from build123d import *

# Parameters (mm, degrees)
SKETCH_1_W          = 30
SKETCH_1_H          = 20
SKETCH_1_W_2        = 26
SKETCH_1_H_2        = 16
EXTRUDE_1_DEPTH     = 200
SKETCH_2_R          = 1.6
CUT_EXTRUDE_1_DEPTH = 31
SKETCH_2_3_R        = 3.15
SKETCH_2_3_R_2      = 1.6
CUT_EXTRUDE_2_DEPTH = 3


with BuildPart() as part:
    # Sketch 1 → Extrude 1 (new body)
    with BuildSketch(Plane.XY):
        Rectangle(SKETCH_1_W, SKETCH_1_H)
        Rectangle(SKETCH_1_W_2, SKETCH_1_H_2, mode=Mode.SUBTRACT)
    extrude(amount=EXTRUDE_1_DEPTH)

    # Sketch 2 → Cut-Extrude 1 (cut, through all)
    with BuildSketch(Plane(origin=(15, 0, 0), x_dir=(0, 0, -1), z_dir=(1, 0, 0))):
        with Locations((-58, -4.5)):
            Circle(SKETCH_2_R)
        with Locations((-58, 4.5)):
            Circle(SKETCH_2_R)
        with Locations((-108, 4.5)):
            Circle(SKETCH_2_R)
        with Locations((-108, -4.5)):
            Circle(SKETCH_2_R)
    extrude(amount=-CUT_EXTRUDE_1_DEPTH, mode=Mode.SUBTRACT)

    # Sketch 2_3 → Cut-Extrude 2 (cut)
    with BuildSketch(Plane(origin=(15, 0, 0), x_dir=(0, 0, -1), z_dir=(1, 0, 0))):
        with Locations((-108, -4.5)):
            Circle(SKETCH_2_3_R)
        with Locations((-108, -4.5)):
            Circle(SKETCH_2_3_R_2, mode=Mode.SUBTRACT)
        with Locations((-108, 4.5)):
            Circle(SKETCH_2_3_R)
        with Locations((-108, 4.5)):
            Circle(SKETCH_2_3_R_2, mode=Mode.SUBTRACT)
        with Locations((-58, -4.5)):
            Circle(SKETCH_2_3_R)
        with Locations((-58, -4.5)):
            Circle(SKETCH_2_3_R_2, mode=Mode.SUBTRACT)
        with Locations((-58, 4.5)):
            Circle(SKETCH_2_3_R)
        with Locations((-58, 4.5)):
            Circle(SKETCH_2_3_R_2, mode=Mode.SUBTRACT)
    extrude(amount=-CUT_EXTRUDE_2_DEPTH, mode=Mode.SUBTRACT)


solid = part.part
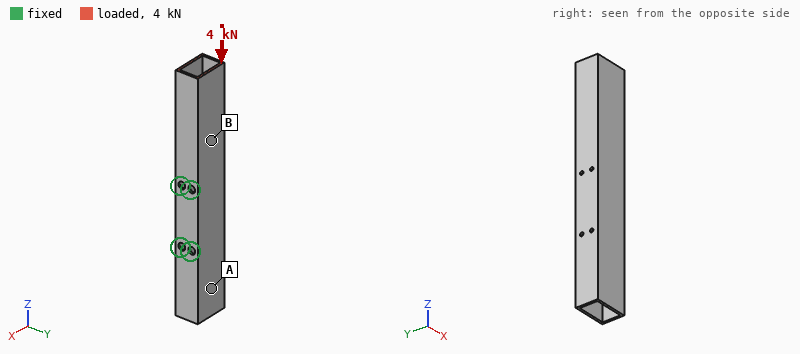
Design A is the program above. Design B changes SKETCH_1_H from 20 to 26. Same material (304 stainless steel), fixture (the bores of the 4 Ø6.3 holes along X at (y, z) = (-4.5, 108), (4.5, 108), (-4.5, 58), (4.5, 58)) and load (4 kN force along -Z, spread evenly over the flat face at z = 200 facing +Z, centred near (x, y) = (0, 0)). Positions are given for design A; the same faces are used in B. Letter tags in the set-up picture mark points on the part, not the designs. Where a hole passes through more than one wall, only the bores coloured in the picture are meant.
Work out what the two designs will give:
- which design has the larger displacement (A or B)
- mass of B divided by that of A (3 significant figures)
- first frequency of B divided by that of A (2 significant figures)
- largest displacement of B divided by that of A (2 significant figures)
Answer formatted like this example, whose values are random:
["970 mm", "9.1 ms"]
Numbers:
["A", "1.99", "1.0", "0.56"]
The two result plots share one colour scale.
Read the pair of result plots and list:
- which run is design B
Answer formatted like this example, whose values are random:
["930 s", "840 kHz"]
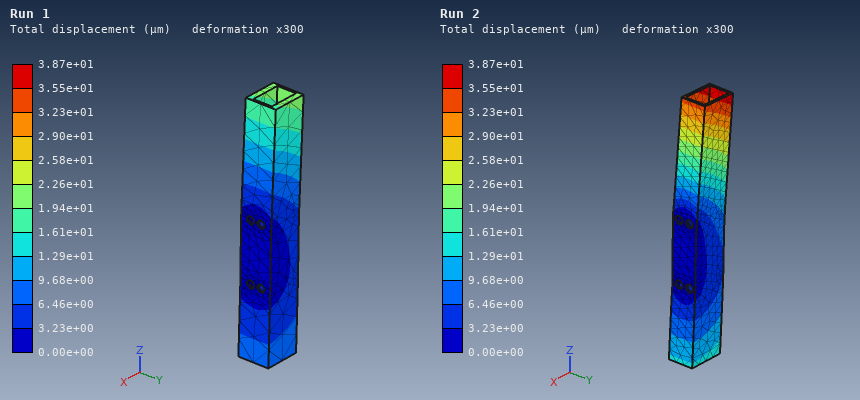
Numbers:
["Run 1"]
